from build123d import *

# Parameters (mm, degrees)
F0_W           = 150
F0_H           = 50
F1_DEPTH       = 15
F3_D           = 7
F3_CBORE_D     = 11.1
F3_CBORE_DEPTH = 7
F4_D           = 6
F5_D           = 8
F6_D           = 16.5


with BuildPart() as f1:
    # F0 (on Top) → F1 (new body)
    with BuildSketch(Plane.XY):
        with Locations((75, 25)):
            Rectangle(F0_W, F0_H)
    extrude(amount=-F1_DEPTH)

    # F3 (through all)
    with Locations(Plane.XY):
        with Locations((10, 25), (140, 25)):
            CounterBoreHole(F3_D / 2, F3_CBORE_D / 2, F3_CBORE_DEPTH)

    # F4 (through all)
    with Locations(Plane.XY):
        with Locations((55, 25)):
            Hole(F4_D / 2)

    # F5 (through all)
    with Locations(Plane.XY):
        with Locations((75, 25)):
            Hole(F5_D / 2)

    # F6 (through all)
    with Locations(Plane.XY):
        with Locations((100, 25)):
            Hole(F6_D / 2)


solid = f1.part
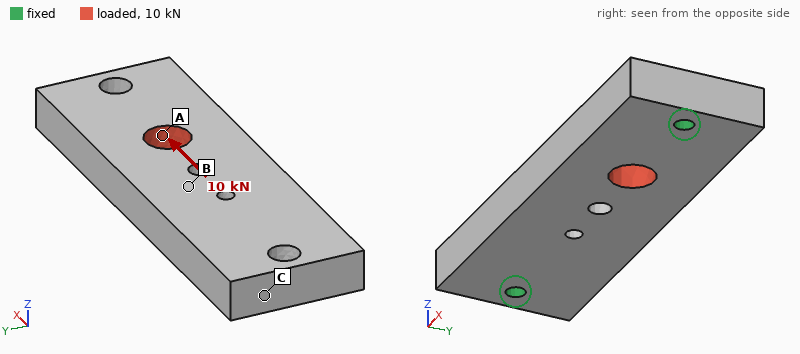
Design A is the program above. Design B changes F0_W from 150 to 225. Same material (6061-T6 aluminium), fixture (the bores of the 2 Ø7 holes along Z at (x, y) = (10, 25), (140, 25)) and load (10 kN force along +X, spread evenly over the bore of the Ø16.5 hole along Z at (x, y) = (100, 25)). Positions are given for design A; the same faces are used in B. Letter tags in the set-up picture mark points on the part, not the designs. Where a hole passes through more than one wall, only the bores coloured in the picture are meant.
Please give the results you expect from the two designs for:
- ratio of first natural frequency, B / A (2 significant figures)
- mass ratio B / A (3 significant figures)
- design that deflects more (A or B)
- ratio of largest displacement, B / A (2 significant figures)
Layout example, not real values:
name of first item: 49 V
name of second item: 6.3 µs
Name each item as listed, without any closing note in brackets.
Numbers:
ratio of first natural frequency, B / A: 0.85
mass ratio B / A: 1.53
design that deflects more: B
ratio of largest displacement, B / A: 1.3
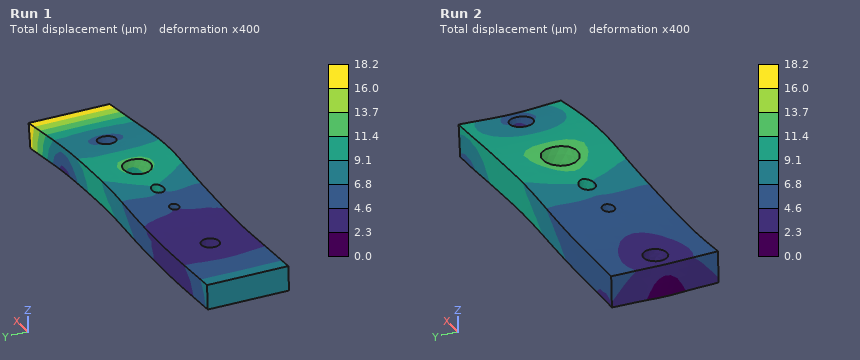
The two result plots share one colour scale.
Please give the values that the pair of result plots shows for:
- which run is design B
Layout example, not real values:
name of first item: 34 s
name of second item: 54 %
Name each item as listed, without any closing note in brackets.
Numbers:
which run is design B: Run 1
